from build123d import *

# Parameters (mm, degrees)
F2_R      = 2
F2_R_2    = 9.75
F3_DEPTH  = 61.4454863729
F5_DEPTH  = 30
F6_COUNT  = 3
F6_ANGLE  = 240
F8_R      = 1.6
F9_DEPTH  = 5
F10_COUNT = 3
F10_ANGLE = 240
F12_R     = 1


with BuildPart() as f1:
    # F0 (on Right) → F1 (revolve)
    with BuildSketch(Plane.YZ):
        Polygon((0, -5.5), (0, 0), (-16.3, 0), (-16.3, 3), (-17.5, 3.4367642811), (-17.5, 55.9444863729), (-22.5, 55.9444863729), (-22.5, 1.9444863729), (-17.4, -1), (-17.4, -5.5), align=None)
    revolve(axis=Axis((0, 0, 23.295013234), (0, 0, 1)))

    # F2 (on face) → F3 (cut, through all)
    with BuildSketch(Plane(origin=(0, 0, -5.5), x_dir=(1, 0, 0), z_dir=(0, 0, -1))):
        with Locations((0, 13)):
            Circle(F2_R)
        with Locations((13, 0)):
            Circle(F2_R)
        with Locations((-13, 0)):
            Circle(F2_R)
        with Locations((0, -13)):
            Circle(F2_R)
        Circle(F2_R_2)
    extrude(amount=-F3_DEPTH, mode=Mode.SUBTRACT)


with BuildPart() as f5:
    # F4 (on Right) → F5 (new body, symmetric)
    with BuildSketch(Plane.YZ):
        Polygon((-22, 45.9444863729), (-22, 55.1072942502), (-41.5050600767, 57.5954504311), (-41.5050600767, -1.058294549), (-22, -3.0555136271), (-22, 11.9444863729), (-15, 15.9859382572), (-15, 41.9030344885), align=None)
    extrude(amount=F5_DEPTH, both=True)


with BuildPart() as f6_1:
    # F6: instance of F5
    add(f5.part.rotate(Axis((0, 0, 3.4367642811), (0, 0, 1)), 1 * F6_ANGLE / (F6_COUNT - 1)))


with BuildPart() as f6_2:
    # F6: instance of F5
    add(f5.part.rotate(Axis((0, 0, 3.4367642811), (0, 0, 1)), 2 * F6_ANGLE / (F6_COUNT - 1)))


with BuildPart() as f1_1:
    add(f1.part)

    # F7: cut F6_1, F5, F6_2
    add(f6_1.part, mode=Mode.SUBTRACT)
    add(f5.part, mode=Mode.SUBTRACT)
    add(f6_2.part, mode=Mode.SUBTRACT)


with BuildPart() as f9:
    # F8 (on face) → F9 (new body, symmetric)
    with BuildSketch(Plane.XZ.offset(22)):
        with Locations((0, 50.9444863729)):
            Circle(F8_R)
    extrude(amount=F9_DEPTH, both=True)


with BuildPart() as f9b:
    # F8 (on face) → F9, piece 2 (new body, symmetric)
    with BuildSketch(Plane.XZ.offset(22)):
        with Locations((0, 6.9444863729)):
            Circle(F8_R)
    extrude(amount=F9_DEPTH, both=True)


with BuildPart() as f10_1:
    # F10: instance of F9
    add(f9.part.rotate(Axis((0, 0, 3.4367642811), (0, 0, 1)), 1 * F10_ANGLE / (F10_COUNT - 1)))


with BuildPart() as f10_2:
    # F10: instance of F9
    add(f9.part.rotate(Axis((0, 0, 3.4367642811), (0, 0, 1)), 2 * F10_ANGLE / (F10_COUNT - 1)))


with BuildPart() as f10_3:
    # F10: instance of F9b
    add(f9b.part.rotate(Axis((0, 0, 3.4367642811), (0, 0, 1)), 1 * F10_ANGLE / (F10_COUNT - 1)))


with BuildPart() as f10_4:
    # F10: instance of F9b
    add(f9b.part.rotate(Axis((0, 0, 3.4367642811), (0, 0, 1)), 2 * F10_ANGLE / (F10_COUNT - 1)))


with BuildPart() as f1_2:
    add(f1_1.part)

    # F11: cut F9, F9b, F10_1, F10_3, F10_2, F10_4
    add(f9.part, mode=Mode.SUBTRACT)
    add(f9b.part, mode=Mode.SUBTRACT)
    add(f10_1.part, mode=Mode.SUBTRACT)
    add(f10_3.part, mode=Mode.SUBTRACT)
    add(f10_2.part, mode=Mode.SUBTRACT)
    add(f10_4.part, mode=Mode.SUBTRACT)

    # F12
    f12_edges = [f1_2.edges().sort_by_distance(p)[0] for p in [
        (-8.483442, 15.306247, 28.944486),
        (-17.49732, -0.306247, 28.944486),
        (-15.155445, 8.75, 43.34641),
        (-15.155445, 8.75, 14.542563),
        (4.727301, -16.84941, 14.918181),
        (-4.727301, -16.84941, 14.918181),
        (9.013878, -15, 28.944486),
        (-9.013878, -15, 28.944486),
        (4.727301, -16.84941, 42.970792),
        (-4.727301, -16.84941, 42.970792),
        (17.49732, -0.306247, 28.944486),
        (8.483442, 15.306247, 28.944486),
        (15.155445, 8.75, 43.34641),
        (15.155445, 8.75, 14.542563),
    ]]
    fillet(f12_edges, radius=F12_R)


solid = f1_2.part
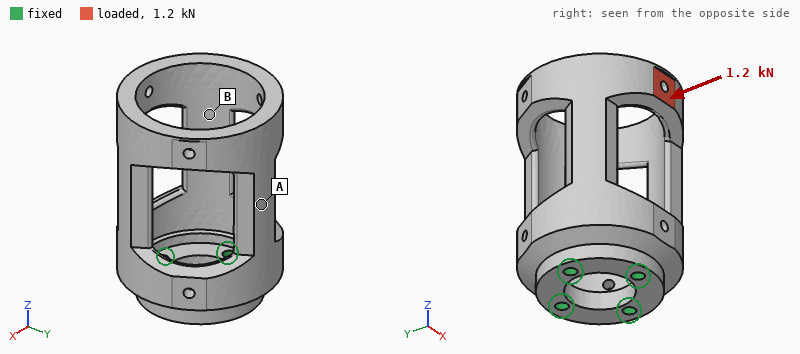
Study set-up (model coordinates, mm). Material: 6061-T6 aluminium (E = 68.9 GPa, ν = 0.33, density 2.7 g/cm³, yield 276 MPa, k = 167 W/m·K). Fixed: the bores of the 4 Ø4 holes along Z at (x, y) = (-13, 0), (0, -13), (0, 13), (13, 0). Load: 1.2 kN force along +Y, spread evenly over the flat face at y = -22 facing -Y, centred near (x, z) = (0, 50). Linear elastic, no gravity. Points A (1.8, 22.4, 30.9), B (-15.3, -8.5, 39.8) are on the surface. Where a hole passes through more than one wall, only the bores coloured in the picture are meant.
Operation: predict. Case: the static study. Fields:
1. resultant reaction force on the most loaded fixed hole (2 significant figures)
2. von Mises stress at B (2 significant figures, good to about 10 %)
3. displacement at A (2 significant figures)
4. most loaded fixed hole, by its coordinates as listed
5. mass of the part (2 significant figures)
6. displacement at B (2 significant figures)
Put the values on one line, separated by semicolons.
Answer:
2.0 kN; 34 MPa; 0.080 mm; (0, -13); 67 g; 0.12 mm
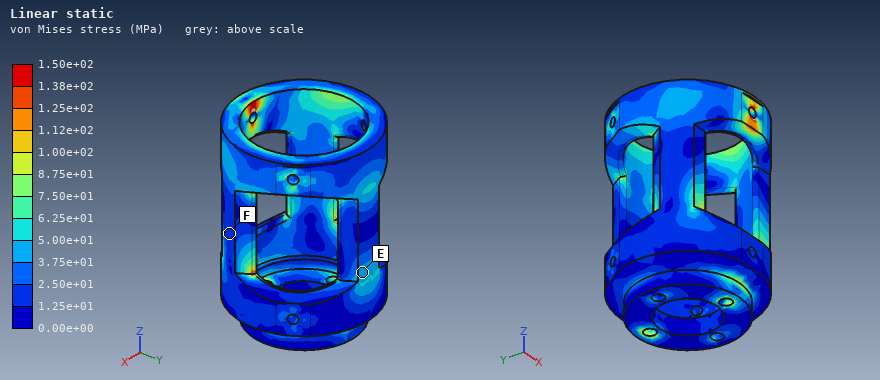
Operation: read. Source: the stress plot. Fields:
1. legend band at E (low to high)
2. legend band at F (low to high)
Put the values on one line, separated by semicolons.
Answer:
3.75e+01 to 5.00e+01 MPa; 1.25e+01 to 2.50e+01 MPa
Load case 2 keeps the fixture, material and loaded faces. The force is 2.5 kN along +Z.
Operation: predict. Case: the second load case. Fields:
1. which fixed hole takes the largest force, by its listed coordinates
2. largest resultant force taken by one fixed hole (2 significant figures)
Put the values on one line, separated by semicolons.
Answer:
(0, -13); 1.8 kN
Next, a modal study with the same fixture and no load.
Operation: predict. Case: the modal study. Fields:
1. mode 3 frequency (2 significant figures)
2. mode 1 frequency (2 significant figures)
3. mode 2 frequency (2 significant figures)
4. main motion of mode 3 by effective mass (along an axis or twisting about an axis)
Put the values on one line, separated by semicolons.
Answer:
5500 Hz; 2800 Hz; 2800 Hz; twisting about Z
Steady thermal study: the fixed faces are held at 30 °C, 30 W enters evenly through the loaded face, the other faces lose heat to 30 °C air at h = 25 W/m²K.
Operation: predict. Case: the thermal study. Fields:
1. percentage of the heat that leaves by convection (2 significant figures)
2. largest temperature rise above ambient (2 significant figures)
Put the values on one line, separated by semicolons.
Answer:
20 %; 66 K
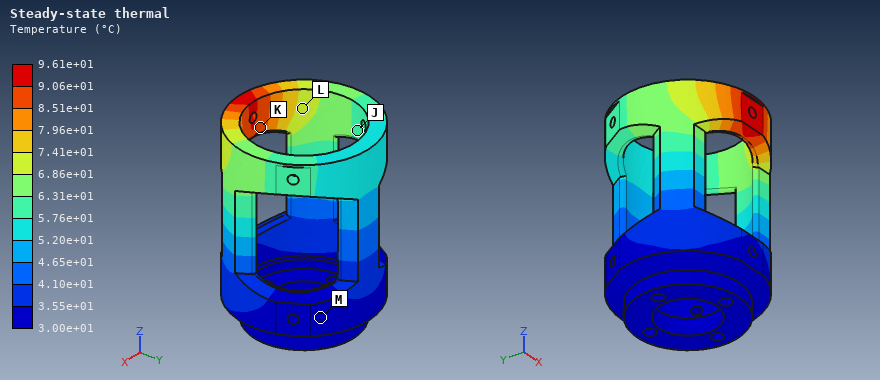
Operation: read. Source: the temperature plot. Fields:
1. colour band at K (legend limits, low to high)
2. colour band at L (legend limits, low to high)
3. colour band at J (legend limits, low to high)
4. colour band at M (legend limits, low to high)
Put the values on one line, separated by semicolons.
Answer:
8.51e+01 to 9.06e+01 °C; 6.86e+01 to 7.41e+01 °C; 5.76e+01 to 6.31e+01 °C; 3.00e+01 to 3.55e+01 °C
